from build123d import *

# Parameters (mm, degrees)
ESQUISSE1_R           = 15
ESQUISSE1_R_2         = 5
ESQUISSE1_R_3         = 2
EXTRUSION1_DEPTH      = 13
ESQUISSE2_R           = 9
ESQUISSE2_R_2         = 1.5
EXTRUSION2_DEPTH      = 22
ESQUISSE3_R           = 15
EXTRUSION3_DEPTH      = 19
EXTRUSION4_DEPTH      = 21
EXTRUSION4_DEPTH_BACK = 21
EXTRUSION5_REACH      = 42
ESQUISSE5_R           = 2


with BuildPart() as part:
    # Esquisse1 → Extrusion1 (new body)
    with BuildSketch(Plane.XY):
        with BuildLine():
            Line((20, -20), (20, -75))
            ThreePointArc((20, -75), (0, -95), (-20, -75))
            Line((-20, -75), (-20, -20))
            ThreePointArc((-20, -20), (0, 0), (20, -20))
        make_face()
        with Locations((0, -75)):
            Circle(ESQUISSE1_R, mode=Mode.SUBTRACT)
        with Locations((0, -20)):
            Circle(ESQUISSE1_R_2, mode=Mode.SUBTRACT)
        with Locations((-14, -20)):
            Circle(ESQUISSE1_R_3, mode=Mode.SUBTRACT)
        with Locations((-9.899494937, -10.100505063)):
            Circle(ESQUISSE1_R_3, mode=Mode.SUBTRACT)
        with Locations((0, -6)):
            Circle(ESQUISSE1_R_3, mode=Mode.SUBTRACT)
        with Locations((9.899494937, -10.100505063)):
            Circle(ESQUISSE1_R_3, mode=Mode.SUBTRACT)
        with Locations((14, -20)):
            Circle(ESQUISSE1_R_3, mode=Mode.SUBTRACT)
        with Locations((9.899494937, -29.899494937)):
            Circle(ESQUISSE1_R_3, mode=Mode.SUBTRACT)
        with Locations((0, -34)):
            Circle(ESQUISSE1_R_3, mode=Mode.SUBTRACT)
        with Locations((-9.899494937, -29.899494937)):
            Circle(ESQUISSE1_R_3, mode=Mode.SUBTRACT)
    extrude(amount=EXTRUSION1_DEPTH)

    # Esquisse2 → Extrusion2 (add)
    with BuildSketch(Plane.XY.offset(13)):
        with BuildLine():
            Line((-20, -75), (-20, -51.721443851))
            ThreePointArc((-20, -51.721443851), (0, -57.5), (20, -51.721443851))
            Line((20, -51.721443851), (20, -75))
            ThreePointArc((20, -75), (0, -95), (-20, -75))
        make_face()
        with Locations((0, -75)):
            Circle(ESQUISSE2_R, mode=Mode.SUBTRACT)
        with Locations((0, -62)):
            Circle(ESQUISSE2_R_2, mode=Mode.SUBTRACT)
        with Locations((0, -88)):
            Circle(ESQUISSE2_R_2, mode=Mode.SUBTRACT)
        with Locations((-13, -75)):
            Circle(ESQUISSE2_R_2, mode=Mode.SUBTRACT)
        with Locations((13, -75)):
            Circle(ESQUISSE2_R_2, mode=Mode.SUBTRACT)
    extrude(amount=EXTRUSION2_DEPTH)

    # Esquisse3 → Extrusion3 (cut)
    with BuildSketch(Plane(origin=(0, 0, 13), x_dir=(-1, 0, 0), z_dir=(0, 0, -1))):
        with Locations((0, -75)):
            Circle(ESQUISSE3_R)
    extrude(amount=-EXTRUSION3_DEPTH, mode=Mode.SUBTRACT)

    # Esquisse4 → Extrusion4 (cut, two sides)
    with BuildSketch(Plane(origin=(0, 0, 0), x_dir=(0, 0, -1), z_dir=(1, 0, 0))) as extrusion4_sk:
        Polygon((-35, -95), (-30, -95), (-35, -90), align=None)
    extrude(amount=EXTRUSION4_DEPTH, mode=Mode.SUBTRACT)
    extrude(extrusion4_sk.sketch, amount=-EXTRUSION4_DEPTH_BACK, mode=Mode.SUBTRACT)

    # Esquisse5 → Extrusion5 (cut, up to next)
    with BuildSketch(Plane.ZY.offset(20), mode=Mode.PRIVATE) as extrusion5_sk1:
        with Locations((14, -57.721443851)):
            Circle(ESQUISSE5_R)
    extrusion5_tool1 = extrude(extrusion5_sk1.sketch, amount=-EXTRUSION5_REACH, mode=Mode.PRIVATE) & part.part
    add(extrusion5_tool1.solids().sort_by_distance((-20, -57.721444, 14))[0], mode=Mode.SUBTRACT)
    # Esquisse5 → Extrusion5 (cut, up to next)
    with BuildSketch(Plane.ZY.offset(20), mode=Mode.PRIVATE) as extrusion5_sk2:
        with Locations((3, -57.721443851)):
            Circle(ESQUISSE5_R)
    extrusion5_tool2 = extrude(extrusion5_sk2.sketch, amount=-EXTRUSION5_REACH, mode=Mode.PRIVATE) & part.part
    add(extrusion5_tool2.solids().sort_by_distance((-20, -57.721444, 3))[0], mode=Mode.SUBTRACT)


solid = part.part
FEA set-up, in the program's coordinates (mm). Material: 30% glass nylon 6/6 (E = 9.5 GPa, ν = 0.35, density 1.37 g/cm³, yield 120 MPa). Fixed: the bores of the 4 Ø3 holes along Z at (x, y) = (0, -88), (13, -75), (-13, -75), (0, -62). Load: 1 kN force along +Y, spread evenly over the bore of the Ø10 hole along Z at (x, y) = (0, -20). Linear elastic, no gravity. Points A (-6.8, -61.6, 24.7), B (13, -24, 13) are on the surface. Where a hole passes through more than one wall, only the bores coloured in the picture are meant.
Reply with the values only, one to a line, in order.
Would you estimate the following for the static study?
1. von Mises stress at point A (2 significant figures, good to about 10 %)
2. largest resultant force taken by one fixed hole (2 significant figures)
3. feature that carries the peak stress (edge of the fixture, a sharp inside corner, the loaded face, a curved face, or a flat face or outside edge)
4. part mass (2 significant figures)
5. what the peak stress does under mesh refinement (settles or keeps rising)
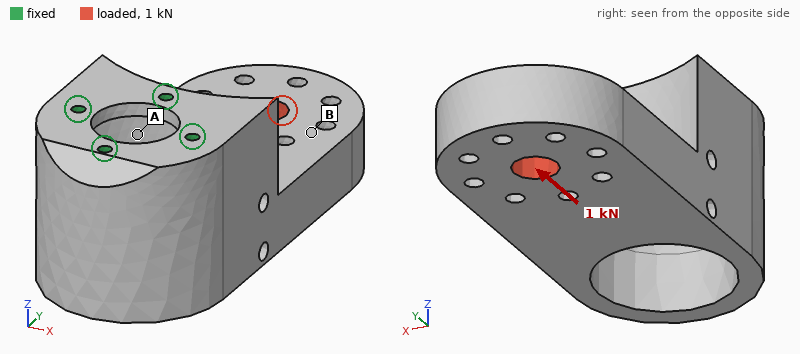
11 MPa
890 N
edge of the fixture
67 g
keeps rising
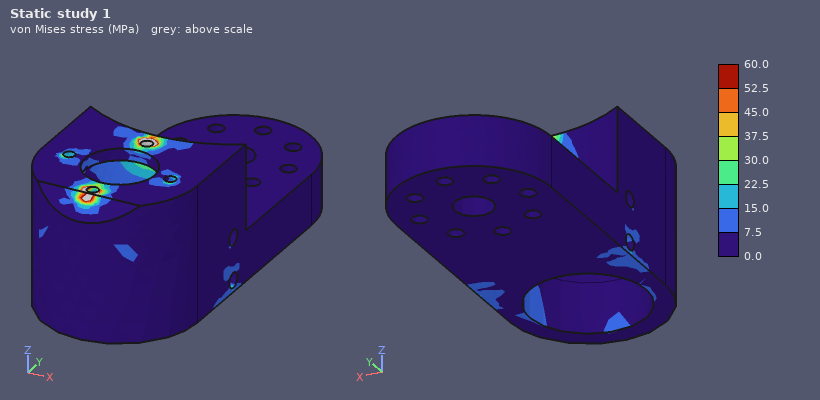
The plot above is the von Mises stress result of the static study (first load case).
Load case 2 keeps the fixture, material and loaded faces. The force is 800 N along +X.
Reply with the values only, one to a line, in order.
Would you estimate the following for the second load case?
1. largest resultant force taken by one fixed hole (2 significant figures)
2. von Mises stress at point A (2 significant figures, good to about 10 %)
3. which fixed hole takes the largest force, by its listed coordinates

1.3 kN
11 MPa
(0, -62)
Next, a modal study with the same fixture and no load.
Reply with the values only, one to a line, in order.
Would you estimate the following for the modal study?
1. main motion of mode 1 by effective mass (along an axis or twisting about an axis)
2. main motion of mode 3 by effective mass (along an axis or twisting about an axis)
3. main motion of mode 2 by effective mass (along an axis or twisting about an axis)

along Z
along Y
along X
